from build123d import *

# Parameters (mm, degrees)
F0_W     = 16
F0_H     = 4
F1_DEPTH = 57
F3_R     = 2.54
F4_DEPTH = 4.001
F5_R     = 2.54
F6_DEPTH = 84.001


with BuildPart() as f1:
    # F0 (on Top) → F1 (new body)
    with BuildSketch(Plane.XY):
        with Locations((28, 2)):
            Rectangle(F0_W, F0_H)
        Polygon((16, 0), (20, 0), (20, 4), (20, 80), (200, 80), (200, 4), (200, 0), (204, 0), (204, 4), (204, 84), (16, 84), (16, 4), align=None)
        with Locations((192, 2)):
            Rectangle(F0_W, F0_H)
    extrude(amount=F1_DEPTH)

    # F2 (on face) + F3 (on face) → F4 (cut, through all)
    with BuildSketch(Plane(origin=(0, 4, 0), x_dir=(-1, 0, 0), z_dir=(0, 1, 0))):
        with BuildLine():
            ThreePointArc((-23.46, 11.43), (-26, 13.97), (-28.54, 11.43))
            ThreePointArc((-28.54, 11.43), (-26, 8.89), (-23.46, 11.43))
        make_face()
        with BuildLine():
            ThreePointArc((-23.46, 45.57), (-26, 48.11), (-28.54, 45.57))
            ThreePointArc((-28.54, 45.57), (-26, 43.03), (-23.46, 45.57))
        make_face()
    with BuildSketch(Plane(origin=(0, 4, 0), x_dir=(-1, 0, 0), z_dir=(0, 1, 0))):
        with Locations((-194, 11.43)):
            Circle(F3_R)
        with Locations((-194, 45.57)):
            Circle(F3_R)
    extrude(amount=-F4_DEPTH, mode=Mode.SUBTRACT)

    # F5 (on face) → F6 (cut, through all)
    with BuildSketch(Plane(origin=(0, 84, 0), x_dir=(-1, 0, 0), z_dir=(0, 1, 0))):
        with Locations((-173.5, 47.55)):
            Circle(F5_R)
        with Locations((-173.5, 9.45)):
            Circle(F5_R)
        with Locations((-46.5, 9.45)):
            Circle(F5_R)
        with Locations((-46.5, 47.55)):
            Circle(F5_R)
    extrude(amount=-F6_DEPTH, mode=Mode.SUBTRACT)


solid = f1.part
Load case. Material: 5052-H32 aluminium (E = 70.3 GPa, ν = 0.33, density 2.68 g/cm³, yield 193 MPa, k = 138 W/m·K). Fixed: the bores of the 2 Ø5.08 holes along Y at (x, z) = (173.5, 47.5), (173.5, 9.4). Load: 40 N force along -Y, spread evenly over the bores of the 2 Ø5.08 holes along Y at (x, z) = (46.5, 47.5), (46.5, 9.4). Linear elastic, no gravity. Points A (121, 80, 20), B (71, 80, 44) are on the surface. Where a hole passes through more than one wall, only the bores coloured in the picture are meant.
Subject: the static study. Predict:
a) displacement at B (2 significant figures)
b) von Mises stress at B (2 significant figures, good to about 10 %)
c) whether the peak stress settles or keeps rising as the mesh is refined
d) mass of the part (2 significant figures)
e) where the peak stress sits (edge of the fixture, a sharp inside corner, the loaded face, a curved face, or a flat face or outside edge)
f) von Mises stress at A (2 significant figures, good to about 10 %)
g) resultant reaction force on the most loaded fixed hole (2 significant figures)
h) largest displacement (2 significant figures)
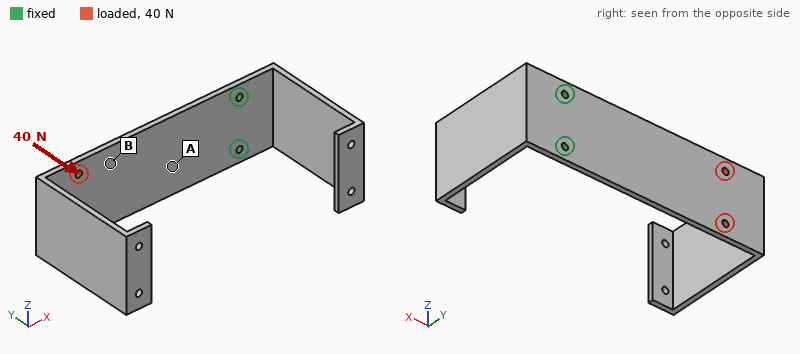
0.90 mm
6.8 MPa
keeps rising
230 g
edge of the fixture
19 MPa
20 N
2.1 mm
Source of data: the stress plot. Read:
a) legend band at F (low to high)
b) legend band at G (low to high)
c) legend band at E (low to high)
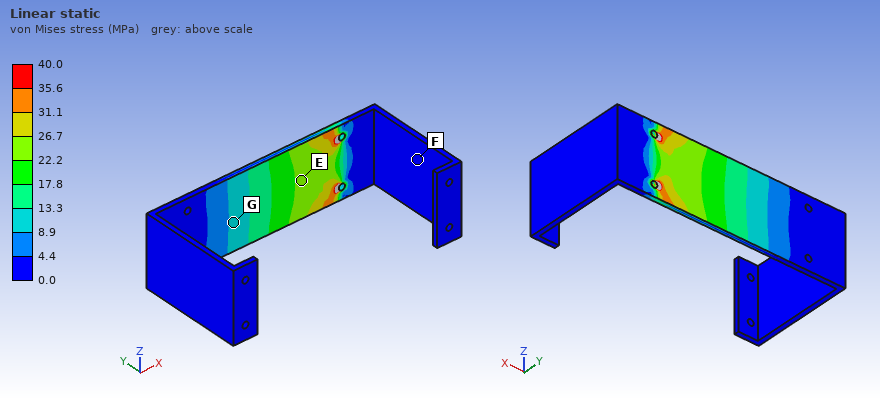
0.0 to 4.4 MPa
8.9 to 13.3 MPa
22.2 to 26.7 MPa
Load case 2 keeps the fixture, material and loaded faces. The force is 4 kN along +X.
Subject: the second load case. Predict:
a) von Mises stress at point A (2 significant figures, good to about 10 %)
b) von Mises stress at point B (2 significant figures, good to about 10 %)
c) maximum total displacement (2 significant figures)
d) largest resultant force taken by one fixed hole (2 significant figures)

18 MPa
18 MPa
37 µm
2.0 kN
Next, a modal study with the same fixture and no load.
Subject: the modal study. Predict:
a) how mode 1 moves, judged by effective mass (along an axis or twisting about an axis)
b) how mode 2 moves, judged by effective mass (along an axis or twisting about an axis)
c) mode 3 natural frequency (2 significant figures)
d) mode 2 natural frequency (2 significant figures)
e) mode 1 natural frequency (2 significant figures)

along Y
along Z
240 Hz
170 Hz
67 Hz
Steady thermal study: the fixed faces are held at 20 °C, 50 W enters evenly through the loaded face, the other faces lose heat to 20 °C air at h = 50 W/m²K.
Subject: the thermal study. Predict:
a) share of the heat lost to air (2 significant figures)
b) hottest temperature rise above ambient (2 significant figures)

84 %
64 K
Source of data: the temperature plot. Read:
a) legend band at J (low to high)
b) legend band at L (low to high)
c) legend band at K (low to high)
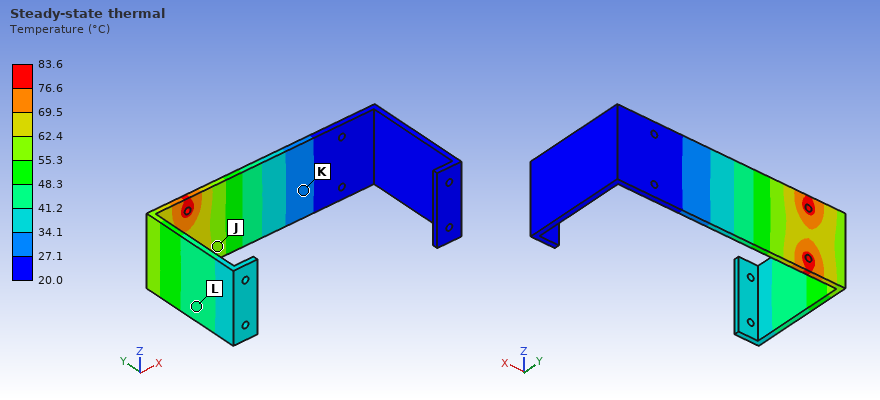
55.3 to 62.4 °C
41.2 to 48.3 °C
27.1 to 34.1 °C
